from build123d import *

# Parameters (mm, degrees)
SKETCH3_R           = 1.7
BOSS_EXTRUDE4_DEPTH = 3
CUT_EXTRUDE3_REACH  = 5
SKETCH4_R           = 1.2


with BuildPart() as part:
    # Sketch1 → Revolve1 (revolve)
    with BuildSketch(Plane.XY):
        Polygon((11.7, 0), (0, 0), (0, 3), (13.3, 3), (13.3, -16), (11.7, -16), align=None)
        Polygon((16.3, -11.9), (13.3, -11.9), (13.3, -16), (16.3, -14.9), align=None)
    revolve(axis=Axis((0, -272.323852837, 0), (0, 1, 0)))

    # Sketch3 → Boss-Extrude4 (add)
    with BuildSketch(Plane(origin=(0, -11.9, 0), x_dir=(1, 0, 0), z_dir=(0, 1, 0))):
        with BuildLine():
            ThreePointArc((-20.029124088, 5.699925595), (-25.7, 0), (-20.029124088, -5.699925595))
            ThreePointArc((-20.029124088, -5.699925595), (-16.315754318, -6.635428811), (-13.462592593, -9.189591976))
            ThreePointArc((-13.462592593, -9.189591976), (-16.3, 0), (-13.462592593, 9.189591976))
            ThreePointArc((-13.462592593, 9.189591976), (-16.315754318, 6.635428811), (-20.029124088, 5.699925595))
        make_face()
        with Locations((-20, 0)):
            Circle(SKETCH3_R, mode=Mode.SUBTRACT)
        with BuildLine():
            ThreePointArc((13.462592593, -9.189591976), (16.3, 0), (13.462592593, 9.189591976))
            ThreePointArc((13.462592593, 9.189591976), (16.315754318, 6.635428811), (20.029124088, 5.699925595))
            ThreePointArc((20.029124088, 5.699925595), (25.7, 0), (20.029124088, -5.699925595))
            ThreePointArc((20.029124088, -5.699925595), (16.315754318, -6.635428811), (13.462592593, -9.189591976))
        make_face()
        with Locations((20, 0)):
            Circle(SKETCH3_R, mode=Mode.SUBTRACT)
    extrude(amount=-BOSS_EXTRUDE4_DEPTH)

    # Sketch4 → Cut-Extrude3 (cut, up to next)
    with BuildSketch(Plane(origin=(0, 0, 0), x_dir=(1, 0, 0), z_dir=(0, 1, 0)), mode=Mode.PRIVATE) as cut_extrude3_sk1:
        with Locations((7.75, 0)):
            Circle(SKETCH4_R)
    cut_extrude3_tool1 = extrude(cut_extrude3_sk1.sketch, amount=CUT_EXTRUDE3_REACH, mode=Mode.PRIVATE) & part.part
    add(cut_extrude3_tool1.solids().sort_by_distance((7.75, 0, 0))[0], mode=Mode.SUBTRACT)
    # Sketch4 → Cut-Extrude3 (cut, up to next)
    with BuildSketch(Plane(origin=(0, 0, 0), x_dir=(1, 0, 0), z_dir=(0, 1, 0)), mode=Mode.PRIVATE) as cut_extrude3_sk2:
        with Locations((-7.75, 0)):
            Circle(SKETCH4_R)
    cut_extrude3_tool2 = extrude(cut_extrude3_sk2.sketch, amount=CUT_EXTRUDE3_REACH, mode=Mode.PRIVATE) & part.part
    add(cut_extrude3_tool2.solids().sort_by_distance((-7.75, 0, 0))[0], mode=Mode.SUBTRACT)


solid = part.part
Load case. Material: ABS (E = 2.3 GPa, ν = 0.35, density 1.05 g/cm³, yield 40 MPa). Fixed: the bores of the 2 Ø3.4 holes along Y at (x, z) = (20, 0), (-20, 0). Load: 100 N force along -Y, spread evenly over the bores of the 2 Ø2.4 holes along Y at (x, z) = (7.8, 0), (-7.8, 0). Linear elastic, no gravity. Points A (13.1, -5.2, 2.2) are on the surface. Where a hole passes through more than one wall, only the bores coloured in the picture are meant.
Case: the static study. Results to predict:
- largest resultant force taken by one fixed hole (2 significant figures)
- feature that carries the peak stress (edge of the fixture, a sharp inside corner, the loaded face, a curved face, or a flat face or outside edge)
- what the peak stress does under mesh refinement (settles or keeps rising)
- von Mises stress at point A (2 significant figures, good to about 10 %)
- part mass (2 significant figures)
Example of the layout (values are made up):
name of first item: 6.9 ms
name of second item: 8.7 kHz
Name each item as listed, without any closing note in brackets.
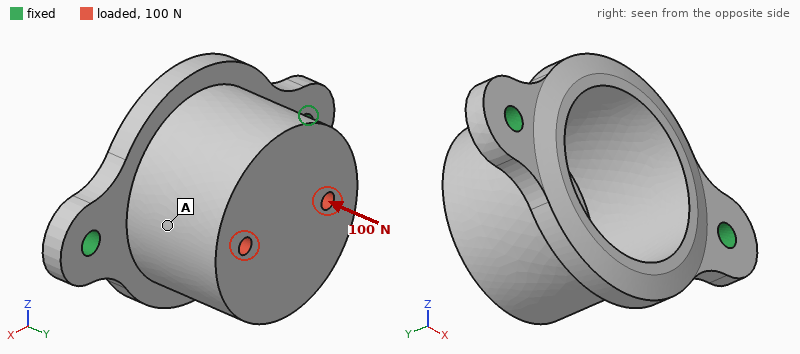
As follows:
largest resultant force taken by one fixed hole: 51 N
feature that carries the peak stress: edge of the fixture
what the peak stress does under mesh refinement: keeps rising
von Mises stress at point A: 2.3 MPa
part mass: 5.5 g
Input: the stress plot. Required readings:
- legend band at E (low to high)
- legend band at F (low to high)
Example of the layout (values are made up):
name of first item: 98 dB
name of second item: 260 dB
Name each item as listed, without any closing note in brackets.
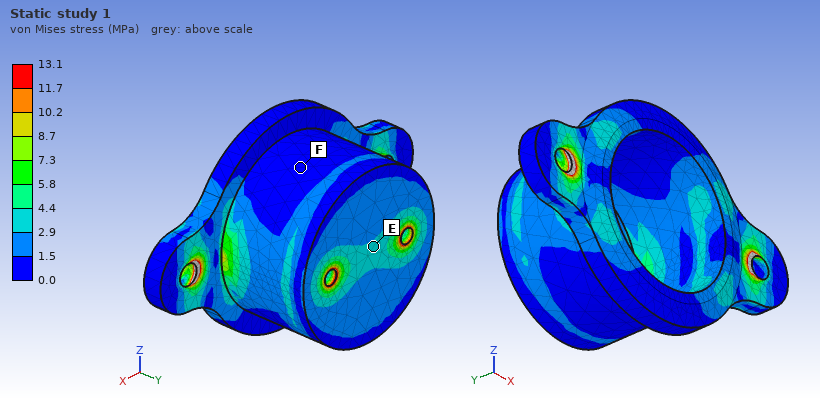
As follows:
legend band at E: 2.9 to 4.4 MPa
legend band at F: 0.0 to 1.5 MPa
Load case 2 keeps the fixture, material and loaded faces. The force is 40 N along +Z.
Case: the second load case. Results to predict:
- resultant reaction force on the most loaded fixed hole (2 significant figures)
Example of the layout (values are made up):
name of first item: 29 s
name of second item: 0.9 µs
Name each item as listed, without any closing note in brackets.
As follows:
resultant reaction force on the most loaded fixed hole: 20 N
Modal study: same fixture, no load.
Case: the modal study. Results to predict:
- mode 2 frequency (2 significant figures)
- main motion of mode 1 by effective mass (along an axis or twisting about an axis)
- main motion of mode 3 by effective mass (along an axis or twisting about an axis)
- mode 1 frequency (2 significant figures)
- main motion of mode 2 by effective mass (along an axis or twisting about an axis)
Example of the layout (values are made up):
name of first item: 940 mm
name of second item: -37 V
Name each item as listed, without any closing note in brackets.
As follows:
mode 2 frequency: 2700 Hz
main motion of mode 1 by effective mass: along Z
main motion of mode 3 by effective mass: along X
mode 1 frequency: 950 Hz
main motion of mode 2 by effective mass: along Y
